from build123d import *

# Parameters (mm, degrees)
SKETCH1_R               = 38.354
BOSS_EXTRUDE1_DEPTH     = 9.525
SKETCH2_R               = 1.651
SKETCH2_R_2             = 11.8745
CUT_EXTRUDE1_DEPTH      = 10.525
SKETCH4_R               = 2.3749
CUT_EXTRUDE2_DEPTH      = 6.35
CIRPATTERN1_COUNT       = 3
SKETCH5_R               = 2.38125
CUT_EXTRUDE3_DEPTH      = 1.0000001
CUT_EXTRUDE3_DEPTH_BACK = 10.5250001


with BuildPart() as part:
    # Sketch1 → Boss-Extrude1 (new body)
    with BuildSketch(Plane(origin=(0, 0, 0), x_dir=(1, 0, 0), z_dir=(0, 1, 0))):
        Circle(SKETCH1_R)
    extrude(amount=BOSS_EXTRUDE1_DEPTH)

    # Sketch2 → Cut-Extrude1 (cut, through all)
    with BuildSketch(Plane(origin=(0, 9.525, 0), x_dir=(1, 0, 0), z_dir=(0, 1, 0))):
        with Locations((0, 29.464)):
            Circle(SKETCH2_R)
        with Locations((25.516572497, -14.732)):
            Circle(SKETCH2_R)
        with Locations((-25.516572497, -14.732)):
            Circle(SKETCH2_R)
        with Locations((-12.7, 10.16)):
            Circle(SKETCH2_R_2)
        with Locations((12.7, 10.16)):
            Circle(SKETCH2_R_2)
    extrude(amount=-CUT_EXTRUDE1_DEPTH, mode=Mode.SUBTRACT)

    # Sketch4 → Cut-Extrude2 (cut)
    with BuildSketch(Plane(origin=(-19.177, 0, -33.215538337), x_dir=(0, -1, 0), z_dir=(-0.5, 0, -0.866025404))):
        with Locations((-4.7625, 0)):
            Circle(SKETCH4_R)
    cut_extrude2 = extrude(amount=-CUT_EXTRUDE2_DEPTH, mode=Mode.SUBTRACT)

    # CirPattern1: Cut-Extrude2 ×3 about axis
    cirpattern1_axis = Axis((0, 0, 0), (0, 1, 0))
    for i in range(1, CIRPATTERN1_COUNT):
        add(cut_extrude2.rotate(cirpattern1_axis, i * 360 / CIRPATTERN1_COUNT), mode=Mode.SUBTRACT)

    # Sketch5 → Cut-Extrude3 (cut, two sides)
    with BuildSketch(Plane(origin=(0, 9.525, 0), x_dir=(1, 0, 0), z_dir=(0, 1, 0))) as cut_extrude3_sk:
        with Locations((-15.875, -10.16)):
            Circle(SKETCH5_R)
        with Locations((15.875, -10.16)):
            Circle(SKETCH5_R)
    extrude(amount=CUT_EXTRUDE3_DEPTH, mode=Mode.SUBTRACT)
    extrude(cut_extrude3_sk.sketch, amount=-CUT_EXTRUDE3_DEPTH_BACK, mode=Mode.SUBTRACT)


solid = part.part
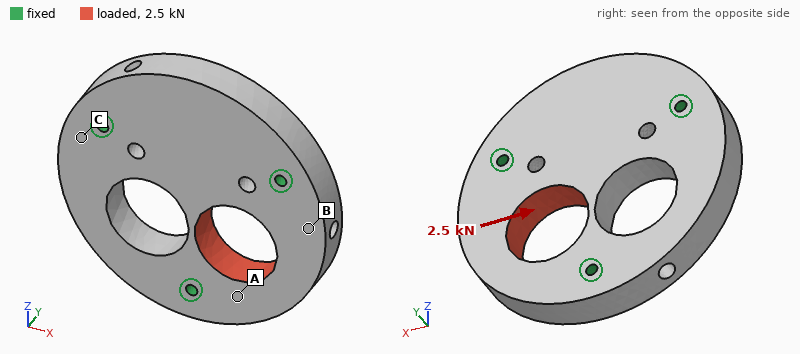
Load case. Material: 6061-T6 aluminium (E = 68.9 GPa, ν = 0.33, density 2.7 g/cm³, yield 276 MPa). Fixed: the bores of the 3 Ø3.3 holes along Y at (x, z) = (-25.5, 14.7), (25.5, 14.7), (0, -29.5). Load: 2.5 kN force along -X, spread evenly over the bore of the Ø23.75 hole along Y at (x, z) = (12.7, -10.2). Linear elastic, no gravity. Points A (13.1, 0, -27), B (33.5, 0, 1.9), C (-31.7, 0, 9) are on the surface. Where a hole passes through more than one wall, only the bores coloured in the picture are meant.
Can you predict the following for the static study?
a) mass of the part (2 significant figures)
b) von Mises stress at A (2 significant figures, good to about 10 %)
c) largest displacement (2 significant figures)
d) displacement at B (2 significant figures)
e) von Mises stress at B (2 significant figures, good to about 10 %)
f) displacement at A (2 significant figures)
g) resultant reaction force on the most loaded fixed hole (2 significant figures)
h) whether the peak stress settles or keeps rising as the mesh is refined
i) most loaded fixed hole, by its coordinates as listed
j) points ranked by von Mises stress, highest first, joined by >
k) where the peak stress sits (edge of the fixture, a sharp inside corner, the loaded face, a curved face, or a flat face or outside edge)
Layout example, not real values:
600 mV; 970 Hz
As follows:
94 g; 8.0 MPa; 7.3 µm; 2.4 µm; 4.1 MPa; 2.0 µm; 1.3 kN; keeps rising; (0, -29.5); A > B > C; edge of the fixture
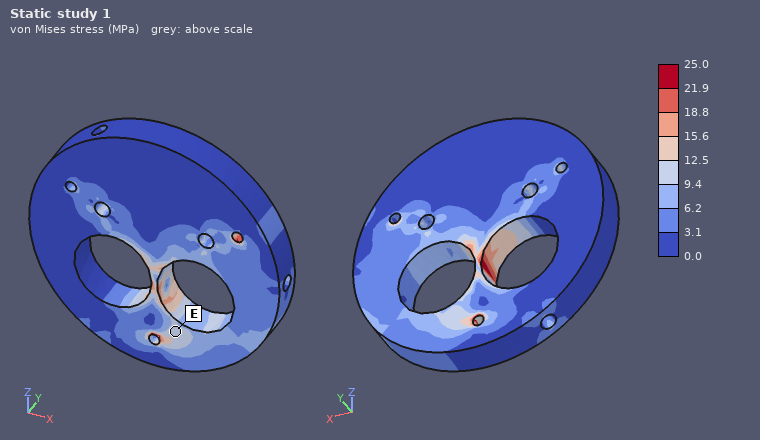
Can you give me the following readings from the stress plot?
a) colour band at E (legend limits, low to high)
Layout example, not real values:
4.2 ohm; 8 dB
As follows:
9.4 to 12.5 MPa
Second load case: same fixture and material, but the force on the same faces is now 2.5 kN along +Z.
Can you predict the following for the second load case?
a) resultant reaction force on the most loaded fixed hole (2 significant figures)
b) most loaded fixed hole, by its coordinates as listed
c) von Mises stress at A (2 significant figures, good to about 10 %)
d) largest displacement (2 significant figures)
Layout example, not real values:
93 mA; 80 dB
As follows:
1.4 kN; (25.5, 14.7); 4.8 MPa; 4.7 µm
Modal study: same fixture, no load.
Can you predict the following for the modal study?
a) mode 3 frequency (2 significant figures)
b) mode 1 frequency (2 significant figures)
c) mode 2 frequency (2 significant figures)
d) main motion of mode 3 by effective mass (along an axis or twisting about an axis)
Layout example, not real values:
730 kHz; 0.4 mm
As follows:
10 kHz; 8600 Hz; 8800 Hz; along Y
